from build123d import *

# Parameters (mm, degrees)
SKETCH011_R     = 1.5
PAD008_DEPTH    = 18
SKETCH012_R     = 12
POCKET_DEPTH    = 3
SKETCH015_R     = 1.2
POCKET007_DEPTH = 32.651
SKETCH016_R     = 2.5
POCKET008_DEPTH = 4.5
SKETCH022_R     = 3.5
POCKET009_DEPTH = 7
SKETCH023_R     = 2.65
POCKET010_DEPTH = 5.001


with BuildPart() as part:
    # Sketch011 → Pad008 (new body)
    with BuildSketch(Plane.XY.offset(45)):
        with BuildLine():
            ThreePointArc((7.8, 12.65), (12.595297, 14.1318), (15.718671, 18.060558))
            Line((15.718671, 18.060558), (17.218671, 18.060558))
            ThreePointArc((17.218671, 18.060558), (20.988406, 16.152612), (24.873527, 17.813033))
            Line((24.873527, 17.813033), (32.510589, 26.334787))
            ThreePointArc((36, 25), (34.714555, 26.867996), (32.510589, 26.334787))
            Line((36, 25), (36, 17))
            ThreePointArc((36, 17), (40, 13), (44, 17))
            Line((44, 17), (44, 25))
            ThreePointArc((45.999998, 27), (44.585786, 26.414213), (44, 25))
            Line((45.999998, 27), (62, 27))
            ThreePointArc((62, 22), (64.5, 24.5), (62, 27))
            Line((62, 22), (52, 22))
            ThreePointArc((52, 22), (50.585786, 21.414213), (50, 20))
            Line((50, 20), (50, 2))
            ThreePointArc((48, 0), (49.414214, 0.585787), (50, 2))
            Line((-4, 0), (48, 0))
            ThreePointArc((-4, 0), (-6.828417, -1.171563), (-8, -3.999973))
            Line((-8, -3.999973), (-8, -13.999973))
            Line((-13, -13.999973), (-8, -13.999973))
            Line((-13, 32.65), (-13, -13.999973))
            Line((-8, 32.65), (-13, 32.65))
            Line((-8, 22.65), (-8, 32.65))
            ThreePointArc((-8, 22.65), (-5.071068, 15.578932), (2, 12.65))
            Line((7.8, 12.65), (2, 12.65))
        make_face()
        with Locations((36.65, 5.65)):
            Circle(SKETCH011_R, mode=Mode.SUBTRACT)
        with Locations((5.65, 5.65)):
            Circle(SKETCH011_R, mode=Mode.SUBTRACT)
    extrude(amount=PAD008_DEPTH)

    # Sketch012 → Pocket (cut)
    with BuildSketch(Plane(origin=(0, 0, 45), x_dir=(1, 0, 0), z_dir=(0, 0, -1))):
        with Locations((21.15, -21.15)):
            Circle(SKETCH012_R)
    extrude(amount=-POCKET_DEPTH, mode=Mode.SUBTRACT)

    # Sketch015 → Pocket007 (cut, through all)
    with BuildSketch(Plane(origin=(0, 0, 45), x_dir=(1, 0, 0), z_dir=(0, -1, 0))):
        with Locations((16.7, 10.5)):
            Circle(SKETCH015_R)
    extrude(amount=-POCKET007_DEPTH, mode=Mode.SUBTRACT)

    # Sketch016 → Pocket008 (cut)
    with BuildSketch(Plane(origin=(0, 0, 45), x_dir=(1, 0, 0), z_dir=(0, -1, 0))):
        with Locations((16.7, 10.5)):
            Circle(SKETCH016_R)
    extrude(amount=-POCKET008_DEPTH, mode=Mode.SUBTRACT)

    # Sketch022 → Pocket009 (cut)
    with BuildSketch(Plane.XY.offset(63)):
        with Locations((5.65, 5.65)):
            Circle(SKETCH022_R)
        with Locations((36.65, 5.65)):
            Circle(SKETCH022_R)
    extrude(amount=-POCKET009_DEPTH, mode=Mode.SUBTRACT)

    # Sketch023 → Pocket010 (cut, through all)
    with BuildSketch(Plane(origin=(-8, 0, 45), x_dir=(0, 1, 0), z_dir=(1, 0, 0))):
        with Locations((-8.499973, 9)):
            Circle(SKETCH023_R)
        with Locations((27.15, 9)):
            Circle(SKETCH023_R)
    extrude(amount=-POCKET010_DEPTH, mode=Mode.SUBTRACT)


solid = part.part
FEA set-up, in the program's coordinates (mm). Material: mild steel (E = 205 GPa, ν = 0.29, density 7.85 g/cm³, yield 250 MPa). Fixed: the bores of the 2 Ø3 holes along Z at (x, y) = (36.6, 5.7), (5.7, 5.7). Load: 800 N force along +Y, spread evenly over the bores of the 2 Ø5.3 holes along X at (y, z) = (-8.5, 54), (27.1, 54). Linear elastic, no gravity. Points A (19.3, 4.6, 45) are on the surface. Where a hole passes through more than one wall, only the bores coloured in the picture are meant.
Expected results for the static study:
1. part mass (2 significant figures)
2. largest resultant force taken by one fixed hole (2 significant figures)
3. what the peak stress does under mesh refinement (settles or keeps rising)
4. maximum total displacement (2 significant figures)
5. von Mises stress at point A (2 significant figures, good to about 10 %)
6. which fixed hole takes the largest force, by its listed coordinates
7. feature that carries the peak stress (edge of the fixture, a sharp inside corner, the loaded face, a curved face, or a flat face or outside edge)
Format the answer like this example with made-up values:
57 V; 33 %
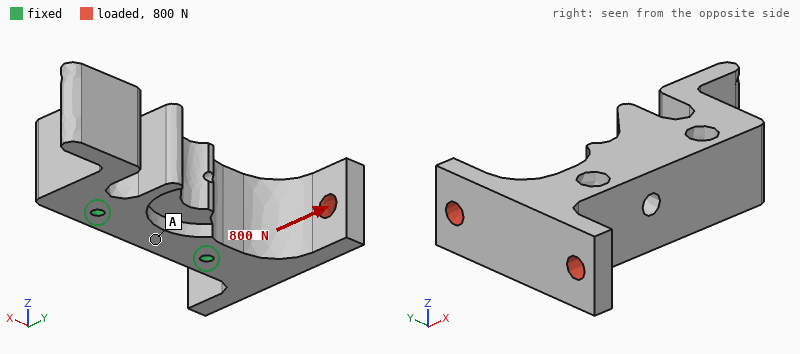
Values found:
180 g; 1.1 kN; keeps rising; 11 µm; 5.8 MPa; (5.7, 5.7); edge of the fixture
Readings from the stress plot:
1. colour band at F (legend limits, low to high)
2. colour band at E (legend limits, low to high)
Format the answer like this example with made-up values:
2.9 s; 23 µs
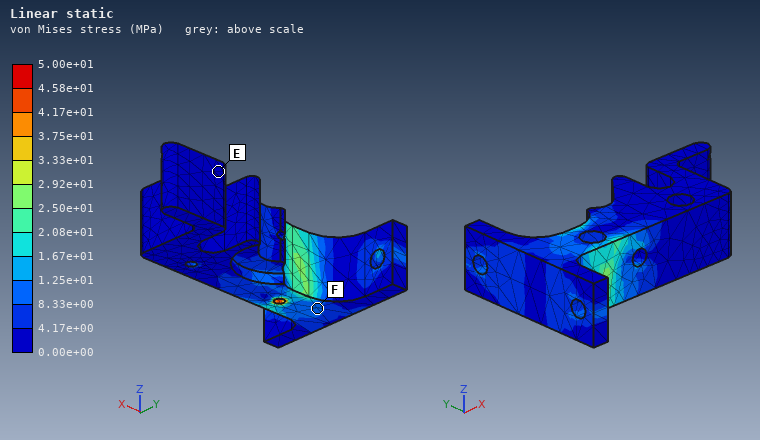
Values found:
8.33e+00 to 1.25e+01 MPa; 0.00e+00 to 4.17e+00 MPa
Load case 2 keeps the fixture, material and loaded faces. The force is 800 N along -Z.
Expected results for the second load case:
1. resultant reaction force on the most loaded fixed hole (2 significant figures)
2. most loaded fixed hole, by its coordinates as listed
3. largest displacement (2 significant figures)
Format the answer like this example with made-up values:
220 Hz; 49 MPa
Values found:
1.0 kN; (5.7, 5.7); 8.5 µm
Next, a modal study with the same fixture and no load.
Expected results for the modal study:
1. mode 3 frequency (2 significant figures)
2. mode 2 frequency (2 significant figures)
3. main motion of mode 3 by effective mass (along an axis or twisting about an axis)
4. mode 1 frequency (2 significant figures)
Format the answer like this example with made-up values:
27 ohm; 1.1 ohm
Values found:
8500 Hz; 7400 Hz; along Z; 6500 Hz
